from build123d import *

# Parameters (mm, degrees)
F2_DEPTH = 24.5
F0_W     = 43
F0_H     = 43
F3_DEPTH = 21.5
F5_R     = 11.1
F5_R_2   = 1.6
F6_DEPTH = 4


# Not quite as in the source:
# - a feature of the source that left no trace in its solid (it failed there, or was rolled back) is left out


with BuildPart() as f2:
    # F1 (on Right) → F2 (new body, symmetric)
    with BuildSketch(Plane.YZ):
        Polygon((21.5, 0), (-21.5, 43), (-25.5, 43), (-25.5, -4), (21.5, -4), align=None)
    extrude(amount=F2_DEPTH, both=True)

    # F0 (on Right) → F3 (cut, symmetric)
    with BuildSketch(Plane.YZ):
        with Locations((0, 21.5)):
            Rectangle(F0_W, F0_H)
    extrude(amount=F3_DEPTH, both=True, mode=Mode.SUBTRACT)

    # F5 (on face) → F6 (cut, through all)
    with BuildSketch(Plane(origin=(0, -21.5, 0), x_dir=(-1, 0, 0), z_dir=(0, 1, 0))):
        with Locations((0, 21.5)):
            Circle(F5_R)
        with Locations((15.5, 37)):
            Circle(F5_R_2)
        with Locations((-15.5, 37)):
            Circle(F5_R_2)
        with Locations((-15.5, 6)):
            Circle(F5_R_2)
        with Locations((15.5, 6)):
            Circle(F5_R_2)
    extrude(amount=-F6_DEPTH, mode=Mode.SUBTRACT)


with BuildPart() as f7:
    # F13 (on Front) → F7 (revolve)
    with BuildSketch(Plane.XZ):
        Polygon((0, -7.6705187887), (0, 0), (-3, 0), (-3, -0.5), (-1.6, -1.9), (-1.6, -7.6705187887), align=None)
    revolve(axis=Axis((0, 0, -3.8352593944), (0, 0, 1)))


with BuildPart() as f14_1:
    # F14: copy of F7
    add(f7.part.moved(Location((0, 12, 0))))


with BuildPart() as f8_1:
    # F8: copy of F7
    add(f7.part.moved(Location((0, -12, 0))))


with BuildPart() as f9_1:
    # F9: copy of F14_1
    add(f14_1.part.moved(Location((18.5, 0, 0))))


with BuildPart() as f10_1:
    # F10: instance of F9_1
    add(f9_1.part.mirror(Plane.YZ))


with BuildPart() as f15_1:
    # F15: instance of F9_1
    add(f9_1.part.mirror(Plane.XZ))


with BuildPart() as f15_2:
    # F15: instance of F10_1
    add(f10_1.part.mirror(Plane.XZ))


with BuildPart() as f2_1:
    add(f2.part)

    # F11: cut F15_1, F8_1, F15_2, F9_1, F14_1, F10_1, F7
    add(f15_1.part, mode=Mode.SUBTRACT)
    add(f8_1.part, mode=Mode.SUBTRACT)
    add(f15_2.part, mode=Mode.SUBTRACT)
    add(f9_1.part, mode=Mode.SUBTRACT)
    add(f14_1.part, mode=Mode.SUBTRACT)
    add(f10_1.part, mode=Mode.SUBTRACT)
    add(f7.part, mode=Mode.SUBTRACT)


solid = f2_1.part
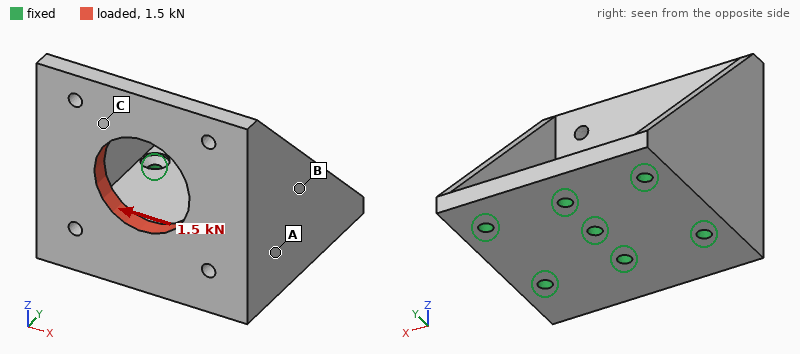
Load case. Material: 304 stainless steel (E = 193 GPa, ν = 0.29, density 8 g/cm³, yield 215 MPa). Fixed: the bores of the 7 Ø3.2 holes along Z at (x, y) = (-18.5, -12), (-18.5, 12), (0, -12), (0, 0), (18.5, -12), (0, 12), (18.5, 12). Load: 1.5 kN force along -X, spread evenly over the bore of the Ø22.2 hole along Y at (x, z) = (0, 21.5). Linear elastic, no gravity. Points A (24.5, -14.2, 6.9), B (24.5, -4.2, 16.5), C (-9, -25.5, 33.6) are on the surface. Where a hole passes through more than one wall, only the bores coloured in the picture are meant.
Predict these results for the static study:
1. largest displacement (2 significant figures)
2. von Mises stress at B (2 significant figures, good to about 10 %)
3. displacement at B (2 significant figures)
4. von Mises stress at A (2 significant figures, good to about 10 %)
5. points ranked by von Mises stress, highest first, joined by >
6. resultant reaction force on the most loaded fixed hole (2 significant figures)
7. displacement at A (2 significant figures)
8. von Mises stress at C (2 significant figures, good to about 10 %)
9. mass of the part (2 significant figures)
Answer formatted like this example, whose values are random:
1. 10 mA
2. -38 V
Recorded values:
1. 31 µm
2. 13 MPa
3. 12 µm
4. 22 MPa
5. A > B > C
6. 1.3 kN
7. 9.1 µm
8. 6.4 MPa
9. 170 g
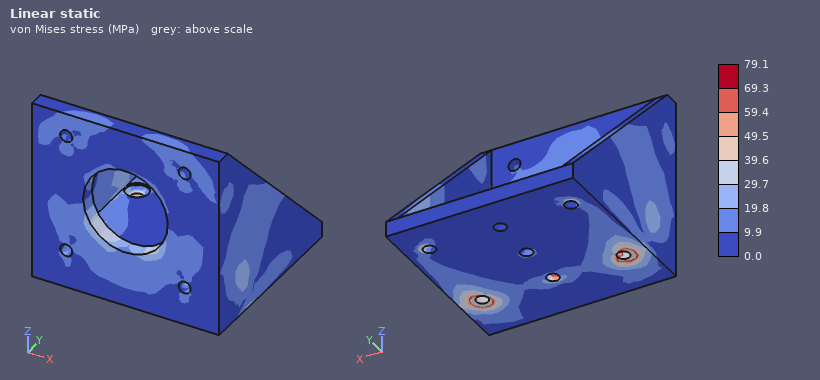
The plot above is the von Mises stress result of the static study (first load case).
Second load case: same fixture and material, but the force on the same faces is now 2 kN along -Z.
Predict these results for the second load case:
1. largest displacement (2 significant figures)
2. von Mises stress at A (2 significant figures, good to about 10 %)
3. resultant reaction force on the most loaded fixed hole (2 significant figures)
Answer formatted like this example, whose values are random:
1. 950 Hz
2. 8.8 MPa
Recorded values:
1. 22 µm
2. 22 MPa
3. 1.3 kN
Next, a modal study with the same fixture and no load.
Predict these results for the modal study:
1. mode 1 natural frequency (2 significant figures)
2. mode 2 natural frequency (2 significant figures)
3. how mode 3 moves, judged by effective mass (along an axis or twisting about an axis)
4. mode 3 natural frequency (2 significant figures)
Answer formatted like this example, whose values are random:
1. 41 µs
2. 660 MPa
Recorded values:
1. 4200 Hz
2. 4300 Hz
3. along Z
4. 7100 Hz
